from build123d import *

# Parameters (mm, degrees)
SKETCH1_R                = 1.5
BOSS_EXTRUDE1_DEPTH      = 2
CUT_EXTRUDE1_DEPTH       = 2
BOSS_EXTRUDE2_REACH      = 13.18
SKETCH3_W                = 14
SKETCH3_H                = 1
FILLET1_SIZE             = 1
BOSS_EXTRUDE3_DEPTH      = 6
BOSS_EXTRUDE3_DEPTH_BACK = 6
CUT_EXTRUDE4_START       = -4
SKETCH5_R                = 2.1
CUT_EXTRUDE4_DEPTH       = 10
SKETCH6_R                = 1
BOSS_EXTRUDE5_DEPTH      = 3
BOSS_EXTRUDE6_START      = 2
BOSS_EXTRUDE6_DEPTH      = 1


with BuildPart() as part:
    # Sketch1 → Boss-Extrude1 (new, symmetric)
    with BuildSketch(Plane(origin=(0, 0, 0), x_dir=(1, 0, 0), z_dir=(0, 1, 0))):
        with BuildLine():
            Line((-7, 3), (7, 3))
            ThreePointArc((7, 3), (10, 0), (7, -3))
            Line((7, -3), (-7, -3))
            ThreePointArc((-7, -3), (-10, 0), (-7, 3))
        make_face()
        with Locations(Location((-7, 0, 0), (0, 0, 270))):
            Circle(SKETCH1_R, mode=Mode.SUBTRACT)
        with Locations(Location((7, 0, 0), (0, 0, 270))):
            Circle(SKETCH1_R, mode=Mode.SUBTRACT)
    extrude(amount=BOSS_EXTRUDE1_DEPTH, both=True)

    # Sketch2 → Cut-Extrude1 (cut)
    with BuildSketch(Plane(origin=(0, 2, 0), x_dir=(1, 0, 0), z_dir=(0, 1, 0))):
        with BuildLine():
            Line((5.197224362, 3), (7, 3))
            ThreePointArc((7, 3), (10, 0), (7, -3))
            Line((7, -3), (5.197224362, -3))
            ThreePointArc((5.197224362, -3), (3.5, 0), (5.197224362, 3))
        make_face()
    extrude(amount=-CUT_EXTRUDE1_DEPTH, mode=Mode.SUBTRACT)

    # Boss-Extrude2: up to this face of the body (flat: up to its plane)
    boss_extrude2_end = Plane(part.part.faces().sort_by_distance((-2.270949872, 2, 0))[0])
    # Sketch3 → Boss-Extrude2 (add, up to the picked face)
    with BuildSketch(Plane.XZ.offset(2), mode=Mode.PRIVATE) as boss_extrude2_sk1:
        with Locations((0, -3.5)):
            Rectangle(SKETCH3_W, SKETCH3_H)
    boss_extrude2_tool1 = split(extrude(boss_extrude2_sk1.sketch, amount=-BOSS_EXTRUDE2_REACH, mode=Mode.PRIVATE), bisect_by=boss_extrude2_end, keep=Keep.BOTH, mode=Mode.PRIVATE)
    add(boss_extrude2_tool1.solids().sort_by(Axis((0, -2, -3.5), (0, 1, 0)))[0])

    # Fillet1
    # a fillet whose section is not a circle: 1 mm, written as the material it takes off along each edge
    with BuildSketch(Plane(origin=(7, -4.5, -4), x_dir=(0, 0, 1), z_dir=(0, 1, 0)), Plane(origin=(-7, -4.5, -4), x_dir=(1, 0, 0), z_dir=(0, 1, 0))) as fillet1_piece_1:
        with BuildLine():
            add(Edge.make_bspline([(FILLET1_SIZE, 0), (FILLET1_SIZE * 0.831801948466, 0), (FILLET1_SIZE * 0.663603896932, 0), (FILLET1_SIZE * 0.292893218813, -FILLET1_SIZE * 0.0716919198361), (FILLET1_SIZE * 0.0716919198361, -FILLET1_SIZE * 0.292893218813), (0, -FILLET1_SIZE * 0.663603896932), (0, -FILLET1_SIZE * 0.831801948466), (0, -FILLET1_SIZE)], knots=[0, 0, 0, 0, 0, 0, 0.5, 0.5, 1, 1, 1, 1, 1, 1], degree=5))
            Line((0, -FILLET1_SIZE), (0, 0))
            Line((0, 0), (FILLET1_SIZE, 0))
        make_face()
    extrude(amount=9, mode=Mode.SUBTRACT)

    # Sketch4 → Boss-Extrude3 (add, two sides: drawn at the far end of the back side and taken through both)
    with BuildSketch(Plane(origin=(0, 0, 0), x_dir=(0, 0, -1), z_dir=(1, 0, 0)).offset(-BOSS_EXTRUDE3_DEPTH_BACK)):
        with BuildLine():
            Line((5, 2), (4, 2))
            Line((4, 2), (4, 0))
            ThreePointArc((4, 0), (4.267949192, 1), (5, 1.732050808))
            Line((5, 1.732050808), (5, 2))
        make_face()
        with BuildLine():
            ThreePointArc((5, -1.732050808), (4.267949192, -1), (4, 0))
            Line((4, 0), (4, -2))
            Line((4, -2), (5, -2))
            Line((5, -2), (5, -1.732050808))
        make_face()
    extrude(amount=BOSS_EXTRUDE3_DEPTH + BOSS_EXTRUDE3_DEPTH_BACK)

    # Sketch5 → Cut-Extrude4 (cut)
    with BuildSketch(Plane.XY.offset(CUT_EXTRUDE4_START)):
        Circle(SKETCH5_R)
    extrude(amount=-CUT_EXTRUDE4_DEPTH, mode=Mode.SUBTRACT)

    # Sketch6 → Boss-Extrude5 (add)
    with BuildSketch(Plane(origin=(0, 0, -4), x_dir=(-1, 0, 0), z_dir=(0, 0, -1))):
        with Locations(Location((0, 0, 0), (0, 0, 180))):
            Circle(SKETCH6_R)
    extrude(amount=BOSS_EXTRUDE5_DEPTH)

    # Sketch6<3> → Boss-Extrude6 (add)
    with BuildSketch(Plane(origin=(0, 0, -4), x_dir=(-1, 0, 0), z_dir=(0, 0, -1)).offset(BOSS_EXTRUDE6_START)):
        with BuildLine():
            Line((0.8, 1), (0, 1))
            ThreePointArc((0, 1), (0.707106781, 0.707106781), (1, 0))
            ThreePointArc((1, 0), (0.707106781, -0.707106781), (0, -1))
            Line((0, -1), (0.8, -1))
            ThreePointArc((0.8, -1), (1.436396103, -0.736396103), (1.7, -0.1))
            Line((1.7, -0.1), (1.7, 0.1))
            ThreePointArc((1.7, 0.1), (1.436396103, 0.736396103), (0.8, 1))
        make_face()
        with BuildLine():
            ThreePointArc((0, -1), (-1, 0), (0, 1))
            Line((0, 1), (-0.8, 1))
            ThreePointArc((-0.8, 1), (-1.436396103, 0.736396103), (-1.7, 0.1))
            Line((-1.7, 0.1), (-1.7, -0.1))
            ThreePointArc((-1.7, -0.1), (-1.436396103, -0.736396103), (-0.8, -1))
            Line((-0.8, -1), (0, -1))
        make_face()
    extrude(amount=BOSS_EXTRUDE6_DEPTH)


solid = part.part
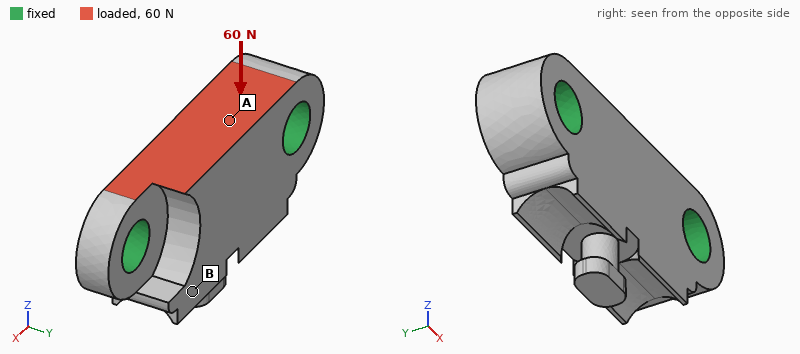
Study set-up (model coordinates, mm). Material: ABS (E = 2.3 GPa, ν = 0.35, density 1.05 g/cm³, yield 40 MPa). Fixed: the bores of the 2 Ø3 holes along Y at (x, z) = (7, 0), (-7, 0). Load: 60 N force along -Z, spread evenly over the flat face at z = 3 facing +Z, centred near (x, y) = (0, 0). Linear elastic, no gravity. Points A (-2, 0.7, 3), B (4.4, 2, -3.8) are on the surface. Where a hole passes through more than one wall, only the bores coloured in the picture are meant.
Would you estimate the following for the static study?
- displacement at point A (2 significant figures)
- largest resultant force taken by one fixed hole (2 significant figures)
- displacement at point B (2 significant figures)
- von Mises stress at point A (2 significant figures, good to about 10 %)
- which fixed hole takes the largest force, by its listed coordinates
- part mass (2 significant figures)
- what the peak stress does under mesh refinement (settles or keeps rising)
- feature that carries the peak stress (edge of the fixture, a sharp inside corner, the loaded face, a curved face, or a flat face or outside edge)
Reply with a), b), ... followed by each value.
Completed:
a) 8.8 µm
b) 34 N
c) 10.0 µm
d) 1.6 MPa
e) (-7, 0)
f) 0.45 g
g) keeps rising
h) edge of the fixture
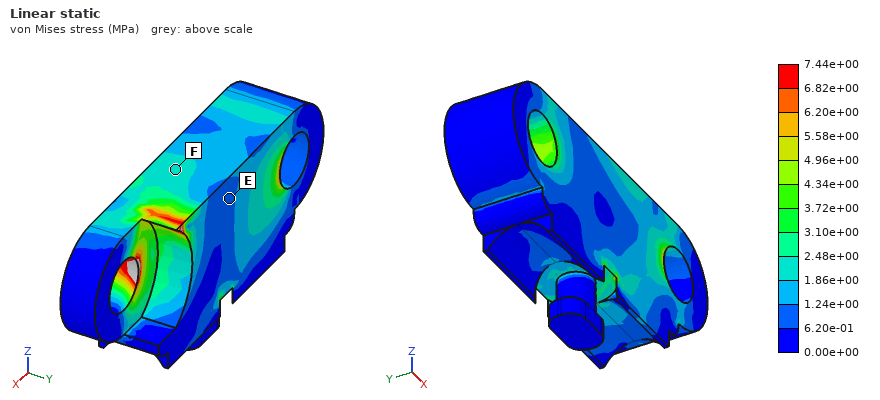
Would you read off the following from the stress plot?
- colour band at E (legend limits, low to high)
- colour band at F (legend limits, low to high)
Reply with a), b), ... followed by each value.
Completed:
a) 6.20e-01 to 1.24e+00 MPa
b) 1.86e+00 to 2.48e+00 MPa
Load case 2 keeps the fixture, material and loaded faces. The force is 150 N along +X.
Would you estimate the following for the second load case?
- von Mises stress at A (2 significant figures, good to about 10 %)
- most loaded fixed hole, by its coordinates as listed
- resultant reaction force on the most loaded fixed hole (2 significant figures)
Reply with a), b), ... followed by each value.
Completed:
a) 5.9 MPa
b) (-7, 0)
c) 100 N
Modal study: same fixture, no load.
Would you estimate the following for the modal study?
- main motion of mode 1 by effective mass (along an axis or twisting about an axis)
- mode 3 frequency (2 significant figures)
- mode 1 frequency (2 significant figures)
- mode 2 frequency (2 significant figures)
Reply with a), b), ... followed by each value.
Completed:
a) along Y
b) 22 kHz
c) 15 kHz
d) 21 kHz
